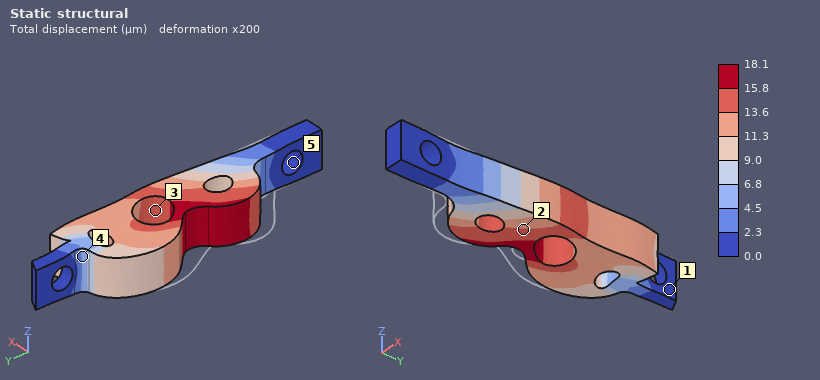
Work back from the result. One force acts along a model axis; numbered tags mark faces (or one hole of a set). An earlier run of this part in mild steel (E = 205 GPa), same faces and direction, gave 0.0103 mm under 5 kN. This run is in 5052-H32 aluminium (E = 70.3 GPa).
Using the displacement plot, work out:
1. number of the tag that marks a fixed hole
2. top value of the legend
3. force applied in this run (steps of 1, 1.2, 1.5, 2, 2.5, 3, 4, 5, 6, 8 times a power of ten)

5
18.1 µm
3 kN
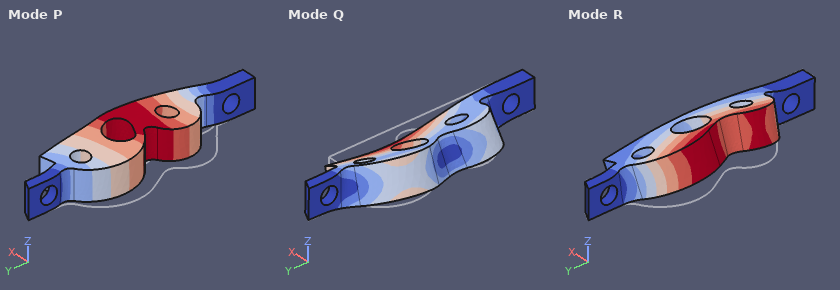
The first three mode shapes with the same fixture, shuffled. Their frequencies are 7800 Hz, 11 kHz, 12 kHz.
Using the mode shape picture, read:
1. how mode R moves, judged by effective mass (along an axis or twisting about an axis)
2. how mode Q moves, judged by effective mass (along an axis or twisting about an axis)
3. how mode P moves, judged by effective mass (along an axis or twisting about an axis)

along Z
along Z
along X
